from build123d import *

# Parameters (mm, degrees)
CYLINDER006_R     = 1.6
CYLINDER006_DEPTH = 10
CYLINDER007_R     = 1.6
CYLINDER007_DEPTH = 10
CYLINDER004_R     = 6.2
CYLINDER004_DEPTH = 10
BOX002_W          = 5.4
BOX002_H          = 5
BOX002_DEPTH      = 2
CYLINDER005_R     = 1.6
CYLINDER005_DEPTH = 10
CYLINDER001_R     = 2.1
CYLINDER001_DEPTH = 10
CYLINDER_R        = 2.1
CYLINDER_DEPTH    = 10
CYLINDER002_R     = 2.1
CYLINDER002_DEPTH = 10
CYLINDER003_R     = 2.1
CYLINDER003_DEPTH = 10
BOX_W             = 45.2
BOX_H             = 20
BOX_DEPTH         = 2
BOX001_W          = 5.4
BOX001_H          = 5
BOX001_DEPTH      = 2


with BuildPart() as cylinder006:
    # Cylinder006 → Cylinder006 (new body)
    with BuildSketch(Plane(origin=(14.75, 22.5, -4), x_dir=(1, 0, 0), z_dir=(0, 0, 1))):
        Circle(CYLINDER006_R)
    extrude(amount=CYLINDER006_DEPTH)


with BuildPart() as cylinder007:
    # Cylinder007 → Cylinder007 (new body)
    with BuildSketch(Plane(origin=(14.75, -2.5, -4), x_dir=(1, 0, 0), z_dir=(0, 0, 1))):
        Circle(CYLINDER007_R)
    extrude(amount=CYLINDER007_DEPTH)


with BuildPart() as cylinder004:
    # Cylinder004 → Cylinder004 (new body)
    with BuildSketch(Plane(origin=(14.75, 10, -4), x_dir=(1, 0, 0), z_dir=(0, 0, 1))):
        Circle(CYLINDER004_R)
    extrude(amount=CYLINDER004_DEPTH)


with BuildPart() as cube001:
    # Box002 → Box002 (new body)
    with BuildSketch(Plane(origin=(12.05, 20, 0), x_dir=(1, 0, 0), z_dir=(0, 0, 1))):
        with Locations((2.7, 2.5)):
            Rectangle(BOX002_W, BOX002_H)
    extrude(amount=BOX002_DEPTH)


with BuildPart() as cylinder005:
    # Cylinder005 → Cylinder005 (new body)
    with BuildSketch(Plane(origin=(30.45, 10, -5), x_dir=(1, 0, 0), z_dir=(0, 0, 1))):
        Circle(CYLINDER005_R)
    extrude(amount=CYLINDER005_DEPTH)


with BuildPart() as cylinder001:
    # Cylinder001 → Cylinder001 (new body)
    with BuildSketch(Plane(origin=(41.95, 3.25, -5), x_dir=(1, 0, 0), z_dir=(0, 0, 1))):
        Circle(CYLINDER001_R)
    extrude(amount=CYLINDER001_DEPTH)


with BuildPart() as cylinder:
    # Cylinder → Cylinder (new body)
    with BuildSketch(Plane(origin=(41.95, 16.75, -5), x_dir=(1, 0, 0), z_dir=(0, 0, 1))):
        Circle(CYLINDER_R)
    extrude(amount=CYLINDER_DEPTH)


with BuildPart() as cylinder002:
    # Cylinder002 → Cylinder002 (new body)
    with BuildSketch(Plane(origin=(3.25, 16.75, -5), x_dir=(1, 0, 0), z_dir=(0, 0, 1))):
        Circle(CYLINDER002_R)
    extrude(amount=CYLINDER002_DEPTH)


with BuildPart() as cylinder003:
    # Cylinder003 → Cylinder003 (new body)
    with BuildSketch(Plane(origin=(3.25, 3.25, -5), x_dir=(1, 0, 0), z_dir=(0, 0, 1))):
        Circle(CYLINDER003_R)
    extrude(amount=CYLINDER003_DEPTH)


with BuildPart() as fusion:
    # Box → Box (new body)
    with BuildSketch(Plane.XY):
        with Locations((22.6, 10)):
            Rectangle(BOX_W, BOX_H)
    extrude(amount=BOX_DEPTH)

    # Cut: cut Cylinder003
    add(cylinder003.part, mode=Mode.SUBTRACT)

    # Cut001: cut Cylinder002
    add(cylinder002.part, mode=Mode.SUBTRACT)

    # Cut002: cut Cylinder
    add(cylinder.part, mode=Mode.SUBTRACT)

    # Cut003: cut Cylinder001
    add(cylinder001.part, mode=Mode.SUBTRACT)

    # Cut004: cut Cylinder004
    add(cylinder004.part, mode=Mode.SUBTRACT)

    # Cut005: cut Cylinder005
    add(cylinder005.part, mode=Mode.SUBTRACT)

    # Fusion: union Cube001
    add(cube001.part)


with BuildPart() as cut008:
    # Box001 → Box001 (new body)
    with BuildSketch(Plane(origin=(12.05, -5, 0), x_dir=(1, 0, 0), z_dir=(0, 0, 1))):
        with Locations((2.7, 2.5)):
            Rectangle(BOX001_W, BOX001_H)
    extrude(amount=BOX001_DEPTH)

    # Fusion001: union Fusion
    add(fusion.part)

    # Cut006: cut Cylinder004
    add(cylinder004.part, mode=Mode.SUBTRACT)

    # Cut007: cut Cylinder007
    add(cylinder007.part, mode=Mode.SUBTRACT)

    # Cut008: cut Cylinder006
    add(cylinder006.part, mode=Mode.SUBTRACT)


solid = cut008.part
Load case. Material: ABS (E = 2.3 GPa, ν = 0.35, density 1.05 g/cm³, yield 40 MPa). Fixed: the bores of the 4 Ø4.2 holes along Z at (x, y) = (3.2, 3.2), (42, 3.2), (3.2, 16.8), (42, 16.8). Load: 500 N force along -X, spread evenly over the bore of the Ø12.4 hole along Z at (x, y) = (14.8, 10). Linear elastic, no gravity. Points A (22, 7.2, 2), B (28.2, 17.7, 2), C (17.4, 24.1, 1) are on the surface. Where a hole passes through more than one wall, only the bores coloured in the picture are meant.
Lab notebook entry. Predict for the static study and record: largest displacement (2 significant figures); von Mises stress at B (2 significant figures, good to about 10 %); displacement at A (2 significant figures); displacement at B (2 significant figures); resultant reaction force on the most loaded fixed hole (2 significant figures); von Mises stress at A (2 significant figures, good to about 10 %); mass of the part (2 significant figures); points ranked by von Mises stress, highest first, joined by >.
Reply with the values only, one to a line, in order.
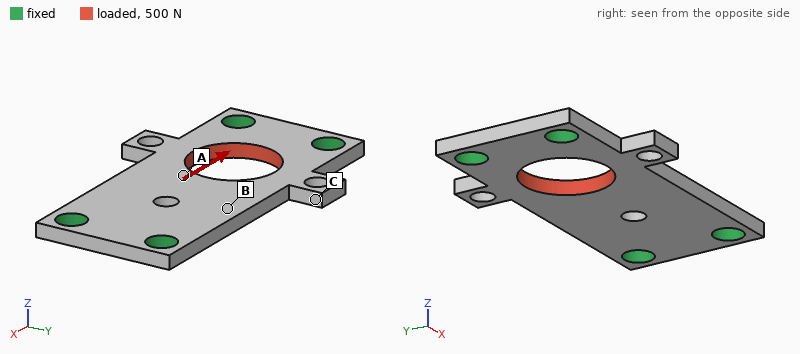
53 µm
4.1 MPa
48 µm
28 µm
160 N
6.7 MPa
1.6 g
A > B > C
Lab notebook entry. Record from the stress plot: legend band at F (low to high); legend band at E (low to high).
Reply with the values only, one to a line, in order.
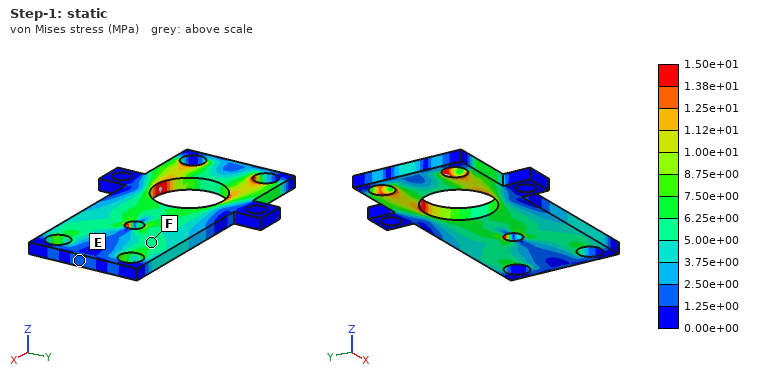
5.00e+00 to 6.25e+00 MPa
1.25e+00 to 2.50e+00 MPa
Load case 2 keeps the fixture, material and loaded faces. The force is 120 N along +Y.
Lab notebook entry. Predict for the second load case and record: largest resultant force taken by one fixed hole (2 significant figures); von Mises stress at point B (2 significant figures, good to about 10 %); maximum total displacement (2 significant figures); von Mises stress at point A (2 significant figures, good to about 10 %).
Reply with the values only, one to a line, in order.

46 N
1.5 MPa
61 µm
2.0 MPa
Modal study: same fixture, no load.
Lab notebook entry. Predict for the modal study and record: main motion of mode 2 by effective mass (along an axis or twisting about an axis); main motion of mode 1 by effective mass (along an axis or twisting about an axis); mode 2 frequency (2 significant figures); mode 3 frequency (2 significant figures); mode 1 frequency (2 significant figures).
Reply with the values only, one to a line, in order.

twisting about X
along Z
2900 Hz
4800 Hz
2200 Hz
